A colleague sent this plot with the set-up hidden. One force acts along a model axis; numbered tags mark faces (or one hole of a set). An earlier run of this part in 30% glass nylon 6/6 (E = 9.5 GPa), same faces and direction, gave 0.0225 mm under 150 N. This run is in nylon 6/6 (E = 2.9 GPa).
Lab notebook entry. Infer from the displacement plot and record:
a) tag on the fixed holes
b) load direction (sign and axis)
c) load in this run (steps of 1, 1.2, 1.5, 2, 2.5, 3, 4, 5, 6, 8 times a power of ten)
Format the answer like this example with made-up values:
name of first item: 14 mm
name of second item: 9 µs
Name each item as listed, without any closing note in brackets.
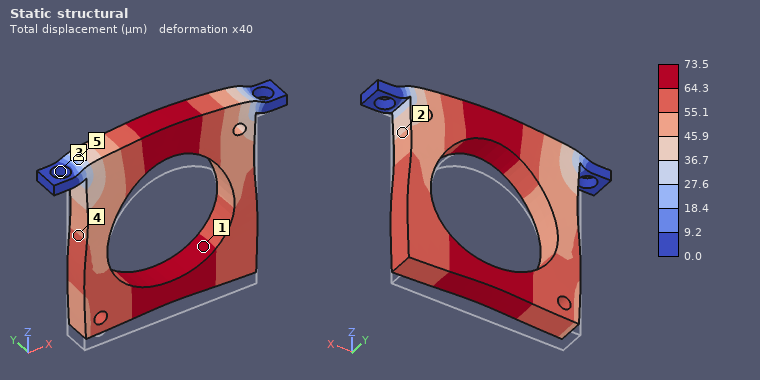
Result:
tag on the fixed holes: 3
load direction: +Z
load in this run: 150 N
